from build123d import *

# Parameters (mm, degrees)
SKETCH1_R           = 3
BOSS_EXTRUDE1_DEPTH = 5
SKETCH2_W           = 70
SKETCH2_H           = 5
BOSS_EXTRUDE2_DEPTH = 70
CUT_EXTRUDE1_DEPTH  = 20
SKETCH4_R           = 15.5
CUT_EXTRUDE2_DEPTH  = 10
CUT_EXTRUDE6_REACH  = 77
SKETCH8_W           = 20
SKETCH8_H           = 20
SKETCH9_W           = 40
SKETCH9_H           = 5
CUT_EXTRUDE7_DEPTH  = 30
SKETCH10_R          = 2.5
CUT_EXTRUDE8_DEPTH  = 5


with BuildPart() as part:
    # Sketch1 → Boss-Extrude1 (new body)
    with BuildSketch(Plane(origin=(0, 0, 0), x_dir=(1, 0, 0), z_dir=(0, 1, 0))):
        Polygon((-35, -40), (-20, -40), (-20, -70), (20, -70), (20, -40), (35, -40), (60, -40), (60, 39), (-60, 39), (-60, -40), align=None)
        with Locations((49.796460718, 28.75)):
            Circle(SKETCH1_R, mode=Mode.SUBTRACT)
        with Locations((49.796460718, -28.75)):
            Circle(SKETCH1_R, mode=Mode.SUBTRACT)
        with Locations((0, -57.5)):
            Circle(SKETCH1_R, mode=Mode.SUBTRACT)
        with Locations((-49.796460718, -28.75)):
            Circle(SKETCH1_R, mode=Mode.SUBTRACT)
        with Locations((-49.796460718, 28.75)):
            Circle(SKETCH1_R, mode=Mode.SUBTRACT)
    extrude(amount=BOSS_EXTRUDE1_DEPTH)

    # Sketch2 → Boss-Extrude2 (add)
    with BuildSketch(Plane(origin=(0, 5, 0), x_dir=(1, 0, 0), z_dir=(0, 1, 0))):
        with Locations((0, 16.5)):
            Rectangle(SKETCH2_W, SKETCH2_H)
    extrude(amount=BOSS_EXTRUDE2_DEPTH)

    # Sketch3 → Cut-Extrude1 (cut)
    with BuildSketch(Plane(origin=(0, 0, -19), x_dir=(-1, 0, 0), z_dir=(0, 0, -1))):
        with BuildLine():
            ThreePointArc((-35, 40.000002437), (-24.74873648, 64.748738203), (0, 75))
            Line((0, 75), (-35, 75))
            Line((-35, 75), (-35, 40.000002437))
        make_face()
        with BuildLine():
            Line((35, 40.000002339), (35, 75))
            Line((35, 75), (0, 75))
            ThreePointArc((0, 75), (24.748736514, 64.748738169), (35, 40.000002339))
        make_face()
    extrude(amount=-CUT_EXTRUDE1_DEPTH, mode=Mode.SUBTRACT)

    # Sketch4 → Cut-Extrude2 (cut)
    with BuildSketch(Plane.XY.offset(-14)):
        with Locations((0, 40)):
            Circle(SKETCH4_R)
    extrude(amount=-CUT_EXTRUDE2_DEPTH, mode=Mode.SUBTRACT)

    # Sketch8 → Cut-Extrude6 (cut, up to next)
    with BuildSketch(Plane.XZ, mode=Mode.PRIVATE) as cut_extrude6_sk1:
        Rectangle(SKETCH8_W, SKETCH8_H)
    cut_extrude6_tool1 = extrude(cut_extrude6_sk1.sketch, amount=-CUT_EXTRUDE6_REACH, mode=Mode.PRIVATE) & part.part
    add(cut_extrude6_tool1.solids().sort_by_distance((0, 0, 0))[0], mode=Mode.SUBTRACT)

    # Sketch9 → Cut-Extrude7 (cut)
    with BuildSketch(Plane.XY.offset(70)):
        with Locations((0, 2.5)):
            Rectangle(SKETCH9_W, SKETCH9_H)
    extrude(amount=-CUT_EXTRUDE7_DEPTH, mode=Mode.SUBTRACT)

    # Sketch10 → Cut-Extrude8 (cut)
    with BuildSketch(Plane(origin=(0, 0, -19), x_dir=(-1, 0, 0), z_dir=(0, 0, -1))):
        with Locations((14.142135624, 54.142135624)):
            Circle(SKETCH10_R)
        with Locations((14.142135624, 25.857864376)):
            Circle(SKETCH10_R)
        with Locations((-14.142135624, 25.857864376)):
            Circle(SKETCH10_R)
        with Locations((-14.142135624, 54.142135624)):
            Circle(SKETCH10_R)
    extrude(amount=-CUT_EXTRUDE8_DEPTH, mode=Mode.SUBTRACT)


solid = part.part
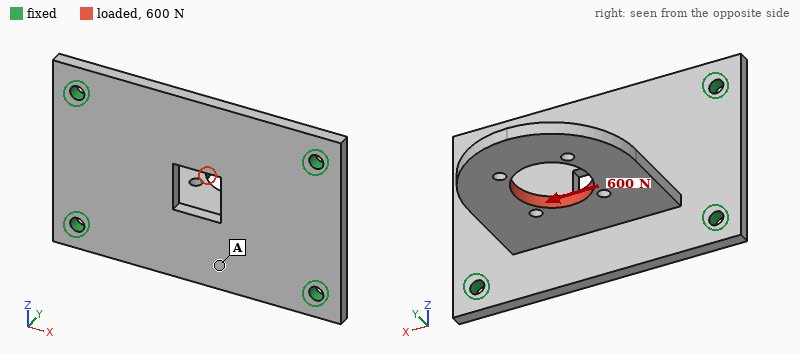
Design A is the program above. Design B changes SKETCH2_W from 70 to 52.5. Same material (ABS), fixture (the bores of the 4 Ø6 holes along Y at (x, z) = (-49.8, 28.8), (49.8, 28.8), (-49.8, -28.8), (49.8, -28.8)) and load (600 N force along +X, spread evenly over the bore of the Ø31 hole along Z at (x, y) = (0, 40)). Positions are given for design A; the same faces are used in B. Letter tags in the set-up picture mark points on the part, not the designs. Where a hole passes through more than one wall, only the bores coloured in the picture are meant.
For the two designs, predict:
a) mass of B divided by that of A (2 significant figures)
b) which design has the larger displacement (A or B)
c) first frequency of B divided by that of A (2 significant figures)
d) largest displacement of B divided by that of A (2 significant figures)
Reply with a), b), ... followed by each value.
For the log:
a) 0.93
b) B
c) 0.89
d) 2.3
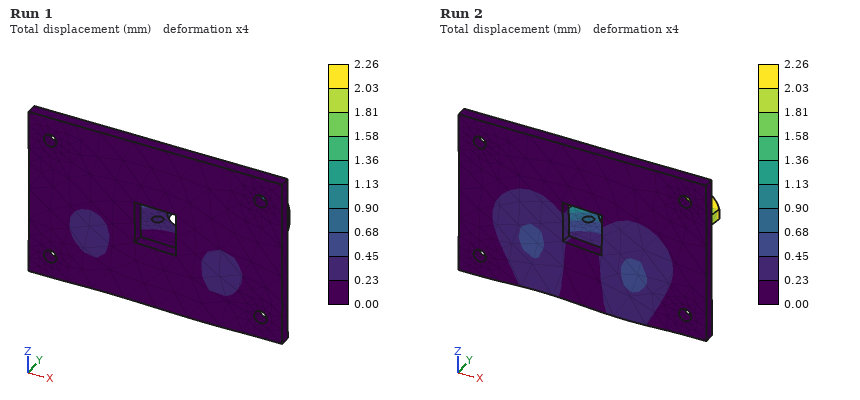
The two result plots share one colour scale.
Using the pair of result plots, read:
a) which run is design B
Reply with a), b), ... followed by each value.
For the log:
a) Run 2
